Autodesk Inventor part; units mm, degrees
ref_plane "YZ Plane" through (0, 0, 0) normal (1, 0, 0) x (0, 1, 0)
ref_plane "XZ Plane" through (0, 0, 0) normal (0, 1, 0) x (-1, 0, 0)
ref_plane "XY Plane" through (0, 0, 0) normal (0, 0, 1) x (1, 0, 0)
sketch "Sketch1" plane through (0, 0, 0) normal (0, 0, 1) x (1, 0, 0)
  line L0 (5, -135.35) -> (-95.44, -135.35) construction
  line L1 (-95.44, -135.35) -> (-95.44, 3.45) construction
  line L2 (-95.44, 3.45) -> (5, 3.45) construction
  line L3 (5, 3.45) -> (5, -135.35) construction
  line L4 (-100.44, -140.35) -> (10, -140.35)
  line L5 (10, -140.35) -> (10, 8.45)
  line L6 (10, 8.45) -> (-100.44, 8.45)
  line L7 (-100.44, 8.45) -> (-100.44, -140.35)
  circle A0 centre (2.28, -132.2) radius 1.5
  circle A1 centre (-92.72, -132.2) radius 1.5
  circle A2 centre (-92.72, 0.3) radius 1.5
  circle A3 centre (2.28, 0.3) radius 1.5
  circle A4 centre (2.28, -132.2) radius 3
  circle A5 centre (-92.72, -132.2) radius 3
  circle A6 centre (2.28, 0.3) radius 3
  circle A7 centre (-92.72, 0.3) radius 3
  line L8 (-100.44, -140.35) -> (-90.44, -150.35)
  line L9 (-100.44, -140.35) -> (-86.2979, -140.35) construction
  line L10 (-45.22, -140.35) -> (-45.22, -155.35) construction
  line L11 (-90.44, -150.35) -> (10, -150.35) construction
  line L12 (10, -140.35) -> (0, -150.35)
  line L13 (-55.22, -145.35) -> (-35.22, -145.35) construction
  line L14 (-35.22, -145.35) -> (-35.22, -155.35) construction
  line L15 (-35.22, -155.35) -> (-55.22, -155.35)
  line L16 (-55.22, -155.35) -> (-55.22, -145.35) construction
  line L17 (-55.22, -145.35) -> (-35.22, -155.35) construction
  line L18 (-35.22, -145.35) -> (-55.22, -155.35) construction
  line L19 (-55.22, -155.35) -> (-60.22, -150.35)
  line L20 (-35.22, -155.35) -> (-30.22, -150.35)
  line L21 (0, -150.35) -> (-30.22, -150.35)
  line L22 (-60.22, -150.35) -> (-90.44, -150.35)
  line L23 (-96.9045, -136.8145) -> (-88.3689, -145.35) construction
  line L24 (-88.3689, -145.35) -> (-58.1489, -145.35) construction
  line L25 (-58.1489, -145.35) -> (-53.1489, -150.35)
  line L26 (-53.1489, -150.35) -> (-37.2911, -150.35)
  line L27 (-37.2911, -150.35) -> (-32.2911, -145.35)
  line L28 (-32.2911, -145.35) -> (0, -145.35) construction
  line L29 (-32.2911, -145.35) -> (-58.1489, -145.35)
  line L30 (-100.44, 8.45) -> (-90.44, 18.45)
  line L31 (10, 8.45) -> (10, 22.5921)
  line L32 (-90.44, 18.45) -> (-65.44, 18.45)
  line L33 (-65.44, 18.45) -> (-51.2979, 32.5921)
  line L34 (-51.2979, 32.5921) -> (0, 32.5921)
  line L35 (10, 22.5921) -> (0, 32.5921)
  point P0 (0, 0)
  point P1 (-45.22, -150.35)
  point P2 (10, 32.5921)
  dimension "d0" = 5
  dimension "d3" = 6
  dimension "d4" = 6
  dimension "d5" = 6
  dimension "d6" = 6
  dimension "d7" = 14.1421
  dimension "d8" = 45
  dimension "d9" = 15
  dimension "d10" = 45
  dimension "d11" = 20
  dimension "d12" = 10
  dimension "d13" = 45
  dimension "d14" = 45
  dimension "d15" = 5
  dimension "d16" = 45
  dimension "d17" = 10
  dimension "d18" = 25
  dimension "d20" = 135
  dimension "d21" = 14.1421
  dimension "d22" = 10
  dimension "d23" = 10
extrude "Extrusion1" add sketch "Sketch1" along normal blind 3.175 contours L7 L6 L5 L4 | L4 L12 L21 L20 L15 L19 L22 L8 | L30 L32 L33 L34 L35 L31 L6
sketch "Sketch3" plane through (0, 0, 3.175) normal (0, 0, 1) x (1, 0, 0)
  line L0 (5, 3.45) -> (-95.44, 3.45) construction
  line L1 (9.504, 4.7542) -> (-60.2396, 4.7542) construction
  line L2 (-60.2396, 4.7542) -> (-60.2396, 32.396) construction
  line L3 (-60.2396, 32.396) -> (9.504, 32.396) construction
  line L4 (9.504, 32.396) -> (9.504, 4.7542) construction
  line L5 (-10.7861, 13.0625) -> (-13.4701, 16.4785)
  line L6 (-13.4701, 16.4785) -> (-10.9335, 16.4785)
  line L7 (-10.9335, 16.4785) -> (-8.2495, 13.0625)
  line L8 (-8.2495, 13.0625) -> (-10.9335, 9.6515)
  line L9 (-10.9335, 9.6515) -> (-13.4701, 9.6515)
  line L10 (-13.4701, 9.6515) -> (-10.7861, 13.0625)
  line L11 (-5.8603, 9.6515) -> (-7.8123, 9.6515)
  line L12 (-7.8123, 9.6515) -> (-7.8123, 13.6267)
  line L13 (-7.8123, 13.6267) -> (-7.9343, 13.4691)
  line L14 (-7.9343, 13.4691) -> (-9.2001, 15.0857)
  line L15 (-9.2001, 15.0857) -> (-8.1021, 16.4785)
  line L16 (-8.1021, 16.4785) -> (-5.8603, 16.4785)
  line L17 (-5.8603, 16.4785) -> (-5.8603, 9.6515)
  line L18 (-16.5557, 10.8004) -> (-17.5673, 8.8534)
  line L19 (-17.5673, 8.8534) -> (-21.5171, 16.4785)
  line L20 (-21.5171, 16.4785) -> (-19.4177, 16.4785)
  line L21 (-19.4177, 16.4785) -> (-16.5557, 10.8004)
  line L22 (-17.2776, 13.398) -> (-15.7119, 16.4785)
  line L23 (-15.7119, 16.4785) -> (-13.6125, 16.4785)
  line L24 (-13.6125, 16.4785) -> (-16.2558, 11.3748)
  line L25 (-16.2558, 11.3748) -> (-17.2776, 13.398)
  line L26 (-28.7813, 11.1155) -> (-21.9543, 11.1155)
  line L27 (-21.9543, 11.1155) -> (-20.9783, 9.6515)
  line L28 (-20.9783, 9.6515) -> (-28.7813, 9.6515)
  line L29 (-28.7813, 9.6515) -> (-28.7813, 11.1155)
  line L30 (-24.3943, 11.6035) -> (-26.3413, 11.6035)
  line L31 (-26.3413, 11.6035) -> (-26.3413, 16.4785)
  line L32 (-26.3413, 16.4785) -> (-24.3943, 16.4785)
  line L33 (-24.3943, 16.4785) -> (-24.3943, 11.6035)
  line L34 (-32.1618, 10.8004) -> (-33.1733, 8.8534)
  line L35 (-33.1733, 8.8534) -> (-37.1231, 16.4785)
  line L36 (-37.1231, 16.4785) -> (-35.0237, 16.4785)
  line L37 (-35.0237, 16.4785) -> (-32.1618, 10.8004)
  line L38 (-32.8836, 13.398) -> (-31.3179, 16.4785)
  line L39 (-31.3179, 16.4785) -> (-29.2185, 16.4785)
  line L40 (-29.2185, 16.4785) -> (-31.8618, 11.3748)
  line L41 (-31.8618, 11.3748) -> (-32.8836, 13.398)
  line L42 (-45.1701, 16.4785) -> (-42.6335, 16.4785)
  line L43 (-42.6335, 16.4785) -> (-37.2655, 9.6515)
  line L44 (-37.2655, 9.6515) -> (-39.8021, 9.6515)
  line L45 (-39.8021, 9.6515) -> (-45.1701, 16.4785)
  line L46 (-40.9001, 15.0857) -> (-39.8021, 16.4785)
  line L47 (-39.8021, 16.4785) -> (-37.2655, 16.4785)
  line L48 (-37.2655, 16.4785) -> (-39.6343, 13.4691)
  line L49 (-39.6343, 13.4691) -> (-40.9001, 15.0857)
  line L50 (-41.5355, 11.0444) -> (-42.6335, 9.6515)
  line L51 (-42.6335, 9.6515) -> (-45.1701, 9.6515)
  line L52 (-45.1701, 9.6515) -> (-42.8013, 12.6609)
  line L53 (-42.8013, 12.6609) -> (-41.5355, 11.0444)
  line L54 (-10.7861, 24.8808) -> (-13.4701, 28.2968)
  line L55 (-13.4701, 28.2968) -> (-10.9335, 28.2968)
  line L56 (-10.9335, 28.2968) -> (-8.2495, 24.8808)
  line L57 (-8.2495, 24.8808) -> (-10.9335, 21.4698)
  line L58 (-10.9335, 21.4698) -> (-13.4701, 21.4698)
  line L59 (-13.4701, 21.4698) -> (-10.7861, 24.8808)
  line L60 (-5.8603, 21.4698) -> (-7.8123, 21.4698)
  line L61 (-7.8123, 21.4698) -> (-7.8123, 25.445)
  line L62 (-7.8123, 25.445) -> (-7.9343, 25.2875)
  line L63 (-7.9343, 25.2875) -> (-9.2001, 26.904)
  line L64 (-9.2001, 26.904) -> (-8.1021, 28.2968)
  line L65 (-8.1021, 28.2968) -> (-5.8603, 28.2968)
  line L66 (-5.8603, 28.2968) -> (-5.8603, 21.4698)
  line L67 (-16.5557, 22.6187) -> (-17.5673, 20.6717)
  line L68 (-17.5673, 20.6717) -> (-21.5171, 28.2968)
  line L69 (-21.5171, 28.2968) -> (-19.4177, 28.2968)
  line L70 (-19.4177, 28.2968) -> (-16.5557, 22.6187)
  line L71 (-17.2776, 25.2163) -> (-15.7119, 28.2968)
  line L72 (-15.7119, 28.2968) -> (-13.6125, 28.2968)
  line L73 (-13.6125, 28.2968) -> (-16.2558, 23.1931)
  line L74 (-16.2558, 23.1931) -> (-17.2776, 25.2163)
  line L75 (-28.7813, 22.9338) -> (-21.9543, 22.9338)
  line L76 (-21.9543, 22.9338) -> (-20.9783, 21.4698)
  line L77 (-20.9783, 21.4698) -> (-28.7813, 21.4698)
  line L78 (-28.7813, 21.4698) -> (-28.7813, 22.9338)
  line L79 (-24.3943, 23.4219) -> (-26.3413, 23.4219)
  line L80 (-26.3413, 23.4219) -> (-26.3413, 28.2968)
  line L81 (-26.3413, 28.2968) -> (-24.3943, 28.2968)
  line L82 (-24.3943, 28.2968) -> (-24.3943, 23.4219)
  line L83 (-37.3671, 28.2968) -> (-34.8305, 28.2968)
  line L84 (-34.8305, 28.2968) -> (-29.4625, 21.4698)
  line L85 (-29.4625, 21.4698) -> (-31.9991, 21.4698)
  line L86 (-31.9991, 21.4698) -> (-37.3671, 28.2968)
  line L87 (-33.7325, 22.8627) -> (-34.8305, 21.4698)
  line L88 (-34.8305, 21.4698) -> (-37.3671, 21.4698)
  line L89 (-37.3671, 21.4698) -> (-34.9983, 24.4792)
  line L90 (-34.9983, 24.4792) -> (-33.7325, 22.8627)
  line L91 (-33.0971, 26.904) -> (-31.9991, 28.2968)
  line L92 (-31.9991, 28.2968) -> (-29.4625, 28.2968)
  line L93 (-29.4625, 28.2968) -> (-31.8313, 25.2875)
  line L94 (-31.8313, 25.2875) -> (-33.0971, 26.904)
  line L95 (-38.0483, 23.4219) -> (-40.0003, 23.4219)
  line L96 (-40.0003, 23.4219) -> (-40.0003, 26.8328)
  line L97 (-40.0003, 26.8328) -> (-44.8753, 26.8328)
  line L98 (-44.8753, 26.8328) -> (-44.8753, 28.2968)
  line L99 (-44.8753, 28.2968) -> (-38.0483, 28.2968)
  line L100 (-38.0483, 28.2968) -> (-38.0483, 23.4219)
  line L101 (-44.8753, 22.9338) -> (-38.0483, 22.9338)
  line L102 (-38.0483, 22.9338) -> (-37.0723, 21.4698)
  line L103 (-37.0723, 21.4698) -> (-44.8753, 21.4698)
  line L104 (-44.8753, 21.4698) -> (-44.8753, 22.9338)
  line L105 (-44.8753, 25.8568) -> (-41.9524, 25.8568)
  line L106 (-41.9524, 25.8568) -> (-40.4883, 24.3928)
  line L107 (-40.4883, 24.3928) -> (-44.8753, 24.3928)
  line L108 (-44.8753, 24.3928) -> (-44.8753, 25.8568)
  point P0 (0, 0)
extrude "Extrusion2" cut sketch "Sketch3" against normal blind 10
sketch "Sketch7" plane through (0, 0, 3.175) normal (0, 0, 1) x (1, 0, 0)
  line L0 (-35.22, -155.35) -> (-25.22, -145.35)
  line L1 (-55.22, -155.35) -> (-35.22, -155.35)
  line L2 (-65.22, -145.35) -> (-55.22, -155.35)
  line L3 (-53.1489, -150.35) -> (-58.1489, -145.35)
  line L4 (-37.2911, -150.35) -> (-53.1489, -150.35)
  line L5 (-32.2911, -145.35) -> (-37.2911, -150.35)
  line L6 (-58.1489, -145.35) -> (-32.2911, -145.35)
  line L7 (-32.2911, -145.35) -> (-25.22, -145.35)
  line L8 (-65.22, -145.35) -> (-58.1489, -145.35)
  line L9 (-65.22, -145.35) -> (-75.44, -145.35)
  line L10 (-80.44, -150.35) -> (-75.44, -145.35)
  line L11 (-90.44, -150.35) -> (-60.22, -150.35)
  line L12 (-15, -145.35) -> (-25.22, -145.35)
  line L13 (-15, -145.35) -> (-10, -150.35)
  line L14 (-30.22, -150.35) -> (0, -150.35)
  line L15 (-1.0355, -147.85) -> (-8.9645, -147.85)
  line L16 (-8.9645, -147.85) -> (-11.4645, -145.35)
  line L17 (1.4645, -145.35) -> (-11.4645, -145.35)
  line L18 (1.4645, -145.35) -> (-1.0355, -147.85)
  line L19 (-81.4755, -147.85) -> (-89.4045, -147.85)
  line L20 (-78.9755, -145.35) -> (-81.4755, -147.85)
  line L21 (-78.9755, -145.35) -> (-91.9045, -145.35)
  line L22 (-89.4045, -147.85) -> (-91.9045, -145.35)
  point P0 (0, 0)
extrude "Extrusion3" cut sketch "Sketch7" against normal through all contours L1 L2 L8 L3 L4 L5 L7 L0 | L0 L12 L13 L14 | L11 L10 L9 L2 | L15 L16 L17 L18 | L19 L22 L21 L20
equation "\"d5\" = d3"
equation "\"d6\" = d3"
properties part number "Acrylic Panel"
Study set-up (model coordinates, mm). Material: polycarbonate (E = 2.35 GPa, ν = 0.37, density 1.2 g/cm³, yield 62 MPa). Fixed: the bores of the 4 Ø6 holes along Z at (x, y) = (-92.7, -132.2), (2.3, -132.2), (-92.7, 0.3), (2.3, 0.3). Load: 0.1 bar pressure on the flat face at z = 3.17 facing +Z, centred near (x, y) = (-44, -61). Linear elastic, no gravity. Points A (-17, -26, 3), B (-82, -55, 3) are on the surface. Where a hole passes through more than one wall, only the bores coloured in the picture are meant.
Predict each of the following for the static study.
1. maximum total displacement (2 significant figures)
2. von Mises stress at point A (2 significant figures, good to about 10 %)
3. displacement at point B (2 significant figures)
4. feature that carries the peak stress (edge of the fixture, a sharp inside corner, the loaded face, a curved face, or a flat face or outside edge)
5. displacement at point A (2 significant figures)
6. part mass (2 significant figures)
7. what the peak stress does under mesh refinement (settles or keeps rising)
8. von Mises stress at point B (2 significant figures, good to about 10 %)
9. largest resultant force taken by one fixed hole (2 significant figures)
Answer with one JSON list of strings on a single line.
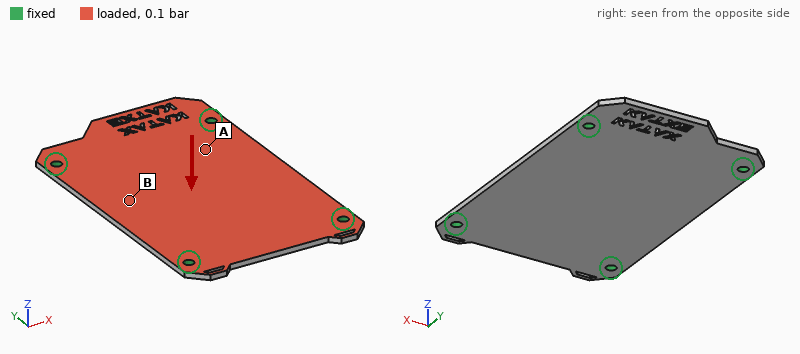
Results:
["1.9 mm", "1.7 MPa", "1.6 mm", "edge of the fixture", "0.97 mm", "71 g", "keeps rising", "4.5 MPa", "51 N"]
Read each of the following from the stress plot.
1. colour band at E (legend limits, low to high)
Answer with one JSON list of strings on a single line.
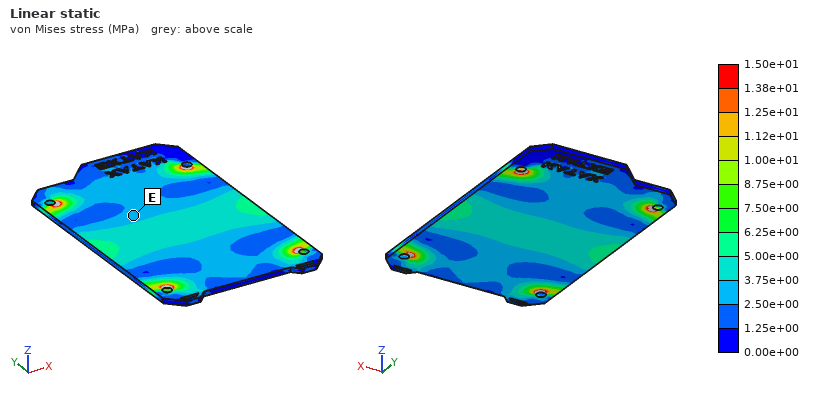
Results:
["2.50e+00 to 3.75e+00 MPa"]
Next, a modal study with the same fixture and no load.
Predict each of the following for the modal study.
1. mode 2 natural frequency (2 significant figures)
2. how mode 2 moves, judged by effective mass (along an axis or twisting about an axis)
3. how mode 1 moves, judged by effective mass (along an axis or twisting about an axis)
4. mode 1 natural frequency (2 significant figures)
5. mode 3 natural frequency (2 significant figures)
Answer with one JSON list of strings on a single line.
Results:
["340 Hz", "twisting about Y", "along Z", "220 Hz", "420 Hz"]
